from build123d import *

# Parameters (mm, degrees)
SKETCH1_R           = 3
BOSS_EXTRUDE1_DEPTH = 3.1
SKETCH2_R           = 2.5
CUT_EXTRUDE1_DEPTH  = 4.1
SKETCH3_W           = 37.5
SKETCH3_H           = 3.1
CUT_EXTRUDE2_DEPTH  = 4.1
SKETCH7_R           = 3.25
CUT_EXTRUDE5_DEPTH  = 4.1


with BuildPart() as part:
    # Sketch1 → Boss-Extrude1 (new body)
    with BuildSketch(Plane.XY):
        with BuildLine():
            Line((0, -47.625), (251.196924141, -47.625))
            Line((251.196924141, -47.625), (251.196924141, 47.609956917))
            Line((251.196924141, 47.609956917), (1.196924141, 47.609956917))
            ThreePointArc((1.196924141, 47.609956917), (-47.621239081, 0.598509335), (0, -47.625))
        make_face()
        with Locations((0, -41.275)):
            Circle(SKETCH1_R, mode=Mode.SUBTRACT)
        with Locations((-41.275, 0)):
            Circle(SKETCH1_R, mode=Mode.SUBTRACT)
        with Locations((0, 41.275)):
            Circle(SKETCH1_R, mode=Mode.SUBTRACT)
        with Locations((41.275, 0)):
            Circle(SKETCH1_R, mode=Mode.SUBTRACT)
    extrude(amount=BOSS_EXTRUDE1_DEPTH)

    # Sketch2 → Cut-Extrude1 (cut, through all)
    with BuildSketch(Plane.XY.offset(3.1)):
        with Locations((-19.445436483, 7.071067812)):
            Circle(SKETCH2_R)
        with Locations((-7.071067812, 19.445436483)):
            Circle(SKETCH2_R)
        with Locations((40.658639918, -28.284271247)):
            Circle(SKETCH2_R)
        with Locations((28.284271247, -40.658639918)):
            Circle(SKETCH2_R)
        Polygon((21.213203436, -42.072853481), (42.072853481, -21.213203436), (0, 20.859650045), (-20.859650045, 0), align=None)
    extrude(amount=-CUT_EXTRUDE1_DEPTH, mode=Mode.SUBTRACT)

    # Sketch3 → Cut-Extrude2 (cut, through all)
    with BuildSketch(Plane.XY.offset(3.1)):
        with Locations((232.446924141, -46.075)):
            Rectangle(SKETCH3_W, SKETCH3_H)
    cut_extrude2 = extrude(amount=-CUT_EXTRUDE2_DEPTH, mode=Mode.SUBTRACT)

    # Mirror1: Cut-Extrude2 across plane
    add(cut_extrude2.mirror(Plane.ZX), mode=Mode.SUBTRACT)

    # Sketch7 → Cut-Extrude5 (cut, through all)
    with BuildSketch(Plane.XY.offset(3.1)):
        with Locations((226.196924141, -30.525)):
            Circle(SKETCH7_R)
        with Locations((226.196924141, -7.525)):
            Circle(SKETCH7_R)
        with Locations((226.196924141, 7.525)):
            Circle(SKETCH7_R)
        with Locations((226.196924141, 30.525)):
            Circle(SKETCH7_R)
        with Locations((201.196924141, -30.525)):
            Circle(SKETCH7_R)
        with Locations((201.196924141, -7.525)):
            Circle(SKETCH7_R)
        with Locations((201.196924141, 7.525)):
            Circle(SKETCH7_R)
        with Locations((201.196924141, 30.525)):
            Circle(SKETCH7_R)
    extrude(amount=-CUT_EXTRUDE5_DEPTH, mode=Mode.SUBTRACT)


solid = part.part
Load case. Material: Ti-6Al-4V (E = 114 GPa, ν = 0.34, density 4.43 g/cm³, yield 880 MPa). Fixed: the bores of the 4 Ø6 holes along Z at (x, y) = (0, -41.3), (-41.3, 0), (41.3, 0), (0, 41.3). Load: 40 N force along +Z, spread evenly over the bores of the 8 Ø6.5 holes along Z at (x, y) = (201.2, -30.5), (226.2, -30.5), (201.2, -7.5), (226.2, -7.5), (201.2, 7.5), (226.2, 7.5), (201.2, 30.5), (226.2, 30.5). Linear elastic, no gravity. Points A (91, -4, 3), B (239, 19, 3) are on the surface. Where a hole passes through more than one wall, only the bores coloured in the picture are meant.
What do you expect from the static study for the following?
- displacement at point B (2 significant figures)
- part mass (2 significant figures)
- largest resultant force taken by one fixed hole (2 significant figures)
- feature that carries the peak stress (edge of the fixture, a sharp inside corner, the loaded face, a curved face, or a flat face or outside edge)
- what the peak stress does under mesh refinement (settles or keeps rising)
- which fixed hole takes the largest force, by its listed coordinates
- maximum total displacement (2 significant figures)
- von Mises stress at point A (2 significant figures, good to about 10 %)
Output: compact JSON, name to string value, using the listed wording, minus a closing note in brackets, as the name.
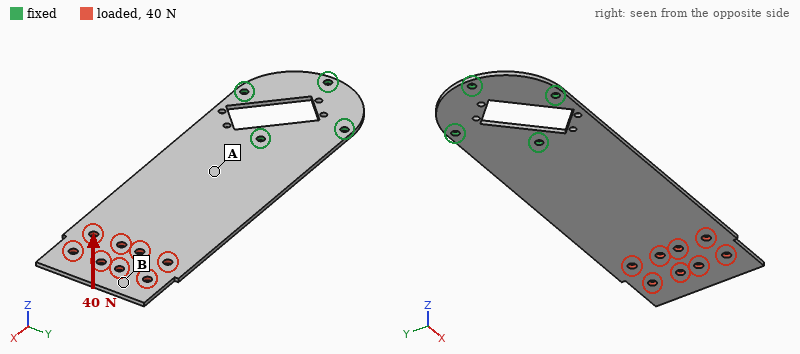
{"displacement at point B": "3.2 mm", "part mass": "340 g", "largest resultant force taken by one fixed hole": "120 N", "feature that carries the peak stress": "edge of the fixture", "what the peak stress does under mesh refinement": "keeps rising", "which fixed hole takes the largest force, by its listed coordinates": "(41.3, 0)", "maximum total displacement": "3.5 mm", "von Mises stress at point A": "28 MPa"}
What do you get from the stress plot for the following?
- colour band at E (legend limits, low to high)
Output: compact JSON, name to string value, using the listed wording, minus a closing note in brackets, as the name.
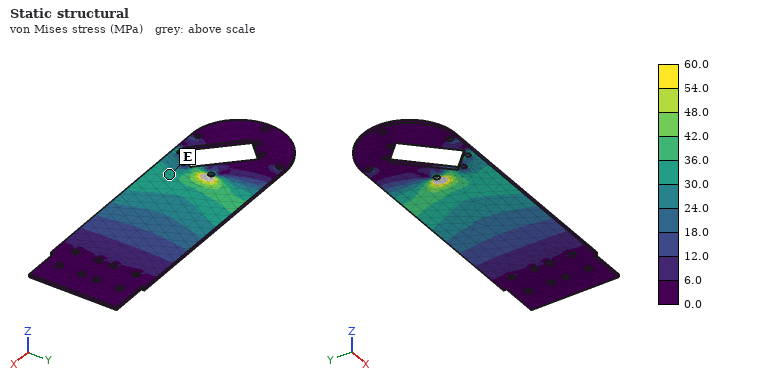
{"colour band at E": "30.0 to 36.0 MPa"}
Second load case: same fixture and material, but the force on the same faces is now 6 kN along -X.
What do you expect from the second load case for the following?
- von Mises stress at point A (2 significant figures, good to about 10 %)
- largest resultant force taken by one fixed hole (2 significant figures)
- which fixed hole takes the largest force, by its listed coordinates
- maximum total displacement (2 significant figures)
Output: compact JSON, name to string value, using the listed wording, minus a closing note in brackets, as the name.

{"von Mises stress at point A": "24 MPa", "largest resultant force taken by one fixed hole": "4.0 kN", "which fixed hole takes the largest force, by its listed coordinates": "(41.3, 0)", "maximum total displacement": "48 µm"}
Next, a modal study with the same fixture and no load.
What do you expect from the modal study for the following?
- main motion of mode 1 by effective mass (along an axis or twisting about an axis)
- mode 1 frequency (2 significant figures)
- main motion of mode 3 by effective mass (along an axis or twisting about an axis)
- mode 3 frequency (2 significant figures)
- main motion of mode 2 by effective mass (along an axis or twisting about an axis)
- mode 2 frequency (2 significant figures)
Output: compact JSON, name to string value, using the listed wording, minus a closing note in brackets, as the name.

{"main motion of mode 1 by effective mass": "along Z", "mode 1 frequency": "58 Hz", "main motion of mode 3 by effective mass": "along Z", "mode 3 frequency": "340 Hz", "main motion of mode 2 by effective mass": "twisting about X", "mode 2 frequency": "240 Hz"}
